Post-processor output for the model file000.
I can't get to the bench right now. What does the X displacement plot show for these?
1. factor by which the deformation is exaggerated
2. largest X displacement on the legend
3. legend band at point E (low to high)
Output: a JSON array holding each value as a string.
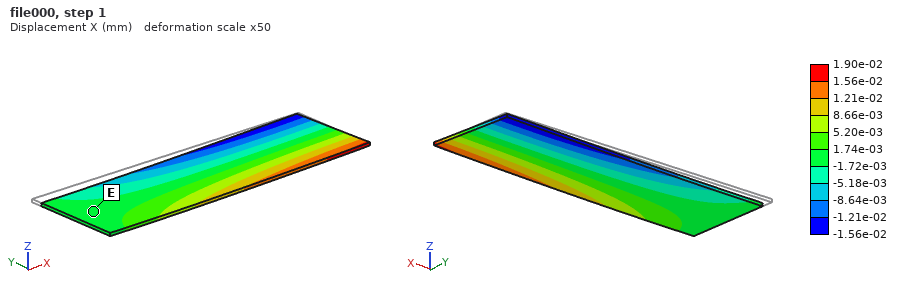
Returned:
["50", "1.90e-02 mm", "-1.72e-03 to 1.74e-03 mm"]
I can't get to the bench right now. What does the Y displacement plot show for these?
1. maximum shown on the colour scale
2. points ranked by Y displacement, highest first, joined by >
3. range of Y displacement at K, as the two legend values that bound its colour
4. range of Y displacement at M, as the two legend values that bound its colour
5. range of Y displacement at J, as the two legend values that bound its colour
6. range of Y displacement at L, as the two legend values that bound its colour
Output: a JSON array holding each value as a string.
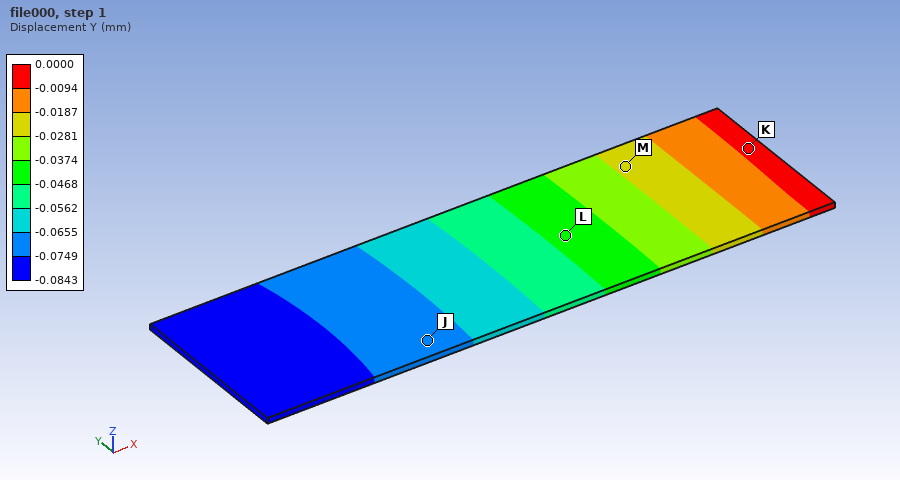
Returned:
["0.0000 mm", "K > M > L > J", "-0.0094 to 0.0000 mm", "-0.0281 to -0.0187 mm", "-0.0749 to -0.0655 mm", "-0.0468 to -0.0374 mm"]
